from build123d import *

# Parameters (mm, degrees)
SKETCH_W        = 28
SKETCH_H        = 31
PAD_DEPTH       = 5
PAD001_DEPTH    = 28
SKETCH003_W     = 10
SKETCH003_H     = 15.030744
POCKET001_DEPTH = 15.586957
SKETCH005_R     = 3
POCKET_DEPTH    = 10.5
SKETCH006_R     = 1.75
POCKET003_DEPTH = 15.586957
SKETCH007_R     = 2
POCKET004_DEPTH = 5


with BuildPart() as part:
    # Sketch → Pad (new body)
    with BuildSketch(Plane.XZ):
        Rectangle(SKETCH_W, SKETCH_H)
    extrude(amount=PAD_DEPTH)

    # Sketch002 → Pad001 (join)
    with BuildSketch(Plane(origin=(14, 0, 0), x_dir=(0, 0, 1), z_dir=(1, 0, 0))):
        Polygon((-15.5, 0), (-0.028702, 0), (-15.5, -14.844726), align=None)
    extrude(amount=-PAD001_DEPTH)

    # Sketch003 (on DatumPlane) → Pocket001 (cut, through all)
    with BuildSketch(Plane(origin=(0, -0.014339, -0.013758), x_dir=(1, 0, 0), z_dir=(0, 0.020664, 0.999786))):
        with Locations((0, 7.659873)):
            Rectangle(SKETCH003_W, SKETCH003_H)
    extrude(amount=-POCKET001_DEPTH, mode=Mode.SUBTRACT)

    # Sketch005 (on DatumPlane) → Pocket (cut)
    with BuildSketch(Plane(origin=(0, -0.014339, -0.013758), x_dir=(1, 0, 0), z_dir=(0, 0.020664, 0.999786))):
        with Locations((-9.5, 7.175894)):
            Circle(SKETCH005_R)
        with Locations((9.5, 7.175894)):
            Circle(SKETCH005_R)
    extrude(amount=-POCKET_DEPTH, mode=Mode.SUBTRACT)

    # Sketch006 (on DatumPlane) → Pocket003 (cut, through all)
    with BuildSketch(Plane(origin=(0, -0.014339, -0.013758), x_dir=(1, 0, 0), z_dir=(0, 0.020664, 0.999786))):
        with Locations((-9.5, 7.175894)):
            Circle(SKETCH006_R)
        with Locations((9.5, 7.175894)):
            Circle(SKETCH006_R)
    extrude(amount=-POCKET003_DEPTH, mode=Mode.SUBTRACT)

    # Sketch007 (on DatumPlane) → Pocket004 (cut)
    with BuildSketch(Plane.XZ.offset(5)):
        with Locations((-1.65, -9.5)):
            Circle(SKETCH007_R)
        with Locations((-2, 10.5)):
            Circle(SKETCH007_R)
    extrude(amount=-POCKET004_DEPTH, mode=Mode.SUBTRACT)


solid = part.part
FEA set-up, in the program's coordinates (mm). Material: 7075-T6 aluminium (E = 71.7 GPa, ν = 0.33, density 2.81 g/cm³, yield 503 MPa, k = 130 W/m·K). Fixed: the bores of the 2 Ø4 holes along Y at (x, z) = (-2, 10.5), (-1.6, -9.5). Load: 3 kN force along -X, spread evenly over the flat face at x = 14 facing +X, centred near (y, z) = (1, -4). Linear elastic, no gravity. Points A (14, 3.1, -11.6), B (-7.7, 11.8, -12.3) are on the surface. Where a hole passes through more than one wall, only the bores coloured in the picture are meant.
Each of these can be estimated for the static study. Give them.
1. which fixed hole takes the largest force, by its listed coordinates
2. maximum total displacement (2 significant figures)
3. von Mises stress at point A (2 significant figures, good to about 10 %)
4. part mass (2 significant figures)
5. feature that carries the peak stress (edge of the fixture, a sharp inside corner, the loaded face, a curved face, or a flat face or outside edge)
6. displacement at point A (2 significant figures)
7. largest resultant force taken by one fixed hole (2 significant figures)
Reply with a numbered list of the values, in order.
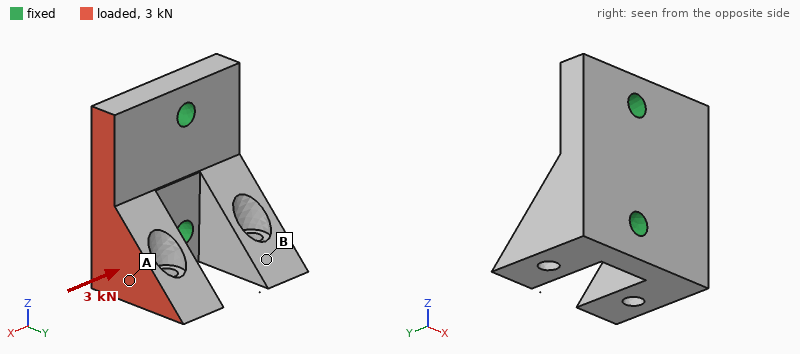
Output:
1. (-1.6, -9.5)
2. 0.13 mm
3. 45 MPa
4. 17 g
5. a flat face or outside edge
6. 0.071 mm
7. 2.2 kN
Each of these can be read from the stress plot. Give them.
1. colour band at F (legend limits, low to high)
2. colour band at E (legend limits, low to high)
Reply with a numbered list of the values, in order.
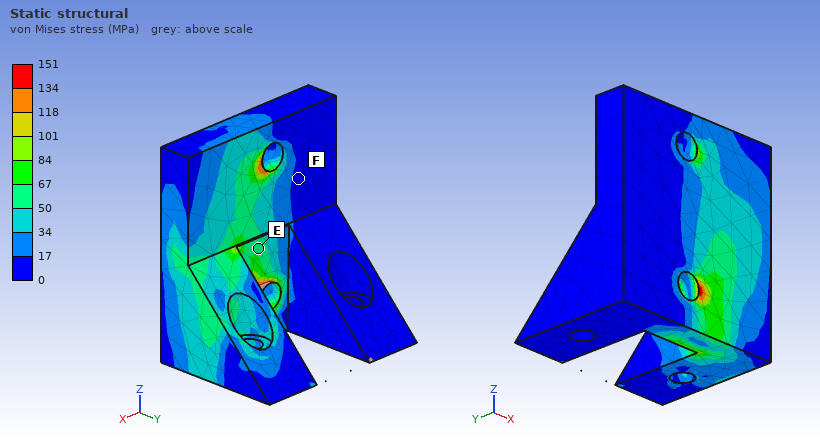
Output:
1. 0 to 17 MPa
2. 50 to 67 MPa
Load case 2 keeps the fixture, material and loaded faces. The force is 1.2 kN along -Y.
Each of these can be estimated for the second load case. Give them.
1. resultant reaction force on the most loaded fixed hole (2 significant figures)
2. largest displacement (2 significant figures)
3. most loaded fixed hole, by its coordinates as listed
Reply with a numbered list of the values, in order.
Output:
1. 850 N
2. 0.14 mm
3. (-1.6, -9.5)
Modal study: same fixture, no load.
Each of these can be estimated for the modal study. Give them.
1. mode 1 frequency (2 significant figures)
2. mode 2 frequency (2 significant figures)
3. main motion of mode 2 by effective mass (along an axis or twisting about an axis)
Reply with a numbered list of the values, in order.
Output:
1. 9700 Hz
2. 14 kHz
3. along Y
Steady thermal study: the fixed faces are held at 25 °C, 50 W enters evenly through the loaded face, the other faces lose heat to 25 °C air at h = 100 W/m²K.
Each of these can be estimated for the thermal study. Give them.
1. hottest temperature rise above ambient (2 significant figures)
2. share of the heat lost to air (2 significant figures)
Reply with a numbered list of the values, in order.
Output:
1. 47 K
2. 7.8 %
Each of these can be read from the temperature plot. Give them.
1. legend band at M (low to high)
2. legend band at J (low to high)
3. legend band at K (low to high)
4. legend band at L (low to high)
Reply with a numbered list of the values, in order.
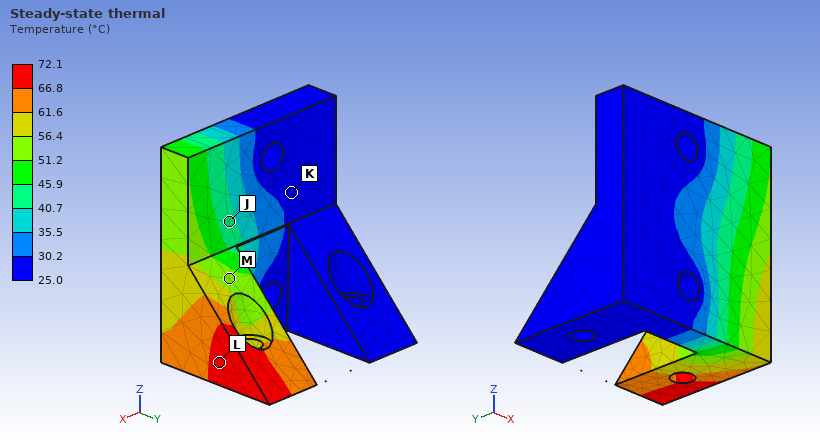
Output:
1. 51.2 to 56.4 °C
2. 40.7 to 45.9 °C
3. 25.0 to 30.2 °C
4. 66.8 to 72.1 °C
